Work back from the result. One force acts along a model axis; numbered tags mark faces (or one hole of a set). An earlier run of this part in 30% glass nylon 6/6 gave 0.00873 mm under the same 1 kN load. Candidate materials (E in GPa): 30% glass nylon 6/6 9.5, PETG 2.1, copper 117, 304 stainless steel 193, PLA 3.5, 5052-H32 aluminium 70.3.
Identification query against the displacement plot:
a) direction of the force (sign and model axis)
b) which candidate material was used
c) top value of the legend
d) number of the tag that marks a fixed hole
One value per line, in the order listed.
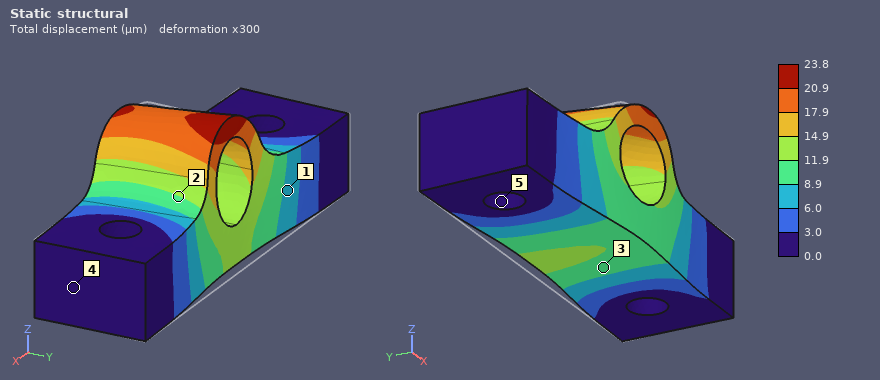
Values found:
-Y
PLA
23.8 µm
5
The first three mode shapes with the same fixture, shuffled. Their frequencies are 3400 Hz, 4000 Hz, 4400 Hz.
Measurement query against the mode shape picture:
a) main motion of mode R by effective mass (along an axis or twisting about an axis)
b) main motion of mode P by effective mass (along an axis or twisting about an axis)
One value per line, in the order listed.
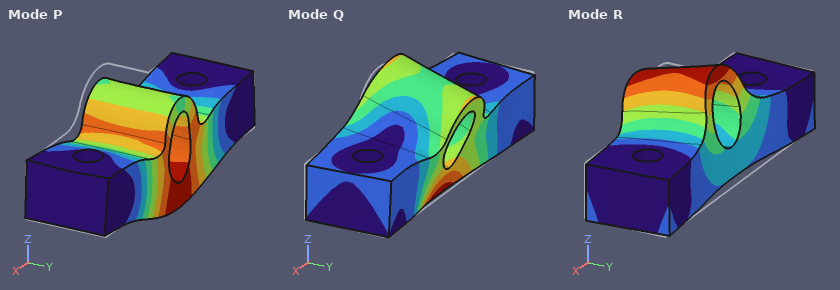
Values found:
along Y
along Z
